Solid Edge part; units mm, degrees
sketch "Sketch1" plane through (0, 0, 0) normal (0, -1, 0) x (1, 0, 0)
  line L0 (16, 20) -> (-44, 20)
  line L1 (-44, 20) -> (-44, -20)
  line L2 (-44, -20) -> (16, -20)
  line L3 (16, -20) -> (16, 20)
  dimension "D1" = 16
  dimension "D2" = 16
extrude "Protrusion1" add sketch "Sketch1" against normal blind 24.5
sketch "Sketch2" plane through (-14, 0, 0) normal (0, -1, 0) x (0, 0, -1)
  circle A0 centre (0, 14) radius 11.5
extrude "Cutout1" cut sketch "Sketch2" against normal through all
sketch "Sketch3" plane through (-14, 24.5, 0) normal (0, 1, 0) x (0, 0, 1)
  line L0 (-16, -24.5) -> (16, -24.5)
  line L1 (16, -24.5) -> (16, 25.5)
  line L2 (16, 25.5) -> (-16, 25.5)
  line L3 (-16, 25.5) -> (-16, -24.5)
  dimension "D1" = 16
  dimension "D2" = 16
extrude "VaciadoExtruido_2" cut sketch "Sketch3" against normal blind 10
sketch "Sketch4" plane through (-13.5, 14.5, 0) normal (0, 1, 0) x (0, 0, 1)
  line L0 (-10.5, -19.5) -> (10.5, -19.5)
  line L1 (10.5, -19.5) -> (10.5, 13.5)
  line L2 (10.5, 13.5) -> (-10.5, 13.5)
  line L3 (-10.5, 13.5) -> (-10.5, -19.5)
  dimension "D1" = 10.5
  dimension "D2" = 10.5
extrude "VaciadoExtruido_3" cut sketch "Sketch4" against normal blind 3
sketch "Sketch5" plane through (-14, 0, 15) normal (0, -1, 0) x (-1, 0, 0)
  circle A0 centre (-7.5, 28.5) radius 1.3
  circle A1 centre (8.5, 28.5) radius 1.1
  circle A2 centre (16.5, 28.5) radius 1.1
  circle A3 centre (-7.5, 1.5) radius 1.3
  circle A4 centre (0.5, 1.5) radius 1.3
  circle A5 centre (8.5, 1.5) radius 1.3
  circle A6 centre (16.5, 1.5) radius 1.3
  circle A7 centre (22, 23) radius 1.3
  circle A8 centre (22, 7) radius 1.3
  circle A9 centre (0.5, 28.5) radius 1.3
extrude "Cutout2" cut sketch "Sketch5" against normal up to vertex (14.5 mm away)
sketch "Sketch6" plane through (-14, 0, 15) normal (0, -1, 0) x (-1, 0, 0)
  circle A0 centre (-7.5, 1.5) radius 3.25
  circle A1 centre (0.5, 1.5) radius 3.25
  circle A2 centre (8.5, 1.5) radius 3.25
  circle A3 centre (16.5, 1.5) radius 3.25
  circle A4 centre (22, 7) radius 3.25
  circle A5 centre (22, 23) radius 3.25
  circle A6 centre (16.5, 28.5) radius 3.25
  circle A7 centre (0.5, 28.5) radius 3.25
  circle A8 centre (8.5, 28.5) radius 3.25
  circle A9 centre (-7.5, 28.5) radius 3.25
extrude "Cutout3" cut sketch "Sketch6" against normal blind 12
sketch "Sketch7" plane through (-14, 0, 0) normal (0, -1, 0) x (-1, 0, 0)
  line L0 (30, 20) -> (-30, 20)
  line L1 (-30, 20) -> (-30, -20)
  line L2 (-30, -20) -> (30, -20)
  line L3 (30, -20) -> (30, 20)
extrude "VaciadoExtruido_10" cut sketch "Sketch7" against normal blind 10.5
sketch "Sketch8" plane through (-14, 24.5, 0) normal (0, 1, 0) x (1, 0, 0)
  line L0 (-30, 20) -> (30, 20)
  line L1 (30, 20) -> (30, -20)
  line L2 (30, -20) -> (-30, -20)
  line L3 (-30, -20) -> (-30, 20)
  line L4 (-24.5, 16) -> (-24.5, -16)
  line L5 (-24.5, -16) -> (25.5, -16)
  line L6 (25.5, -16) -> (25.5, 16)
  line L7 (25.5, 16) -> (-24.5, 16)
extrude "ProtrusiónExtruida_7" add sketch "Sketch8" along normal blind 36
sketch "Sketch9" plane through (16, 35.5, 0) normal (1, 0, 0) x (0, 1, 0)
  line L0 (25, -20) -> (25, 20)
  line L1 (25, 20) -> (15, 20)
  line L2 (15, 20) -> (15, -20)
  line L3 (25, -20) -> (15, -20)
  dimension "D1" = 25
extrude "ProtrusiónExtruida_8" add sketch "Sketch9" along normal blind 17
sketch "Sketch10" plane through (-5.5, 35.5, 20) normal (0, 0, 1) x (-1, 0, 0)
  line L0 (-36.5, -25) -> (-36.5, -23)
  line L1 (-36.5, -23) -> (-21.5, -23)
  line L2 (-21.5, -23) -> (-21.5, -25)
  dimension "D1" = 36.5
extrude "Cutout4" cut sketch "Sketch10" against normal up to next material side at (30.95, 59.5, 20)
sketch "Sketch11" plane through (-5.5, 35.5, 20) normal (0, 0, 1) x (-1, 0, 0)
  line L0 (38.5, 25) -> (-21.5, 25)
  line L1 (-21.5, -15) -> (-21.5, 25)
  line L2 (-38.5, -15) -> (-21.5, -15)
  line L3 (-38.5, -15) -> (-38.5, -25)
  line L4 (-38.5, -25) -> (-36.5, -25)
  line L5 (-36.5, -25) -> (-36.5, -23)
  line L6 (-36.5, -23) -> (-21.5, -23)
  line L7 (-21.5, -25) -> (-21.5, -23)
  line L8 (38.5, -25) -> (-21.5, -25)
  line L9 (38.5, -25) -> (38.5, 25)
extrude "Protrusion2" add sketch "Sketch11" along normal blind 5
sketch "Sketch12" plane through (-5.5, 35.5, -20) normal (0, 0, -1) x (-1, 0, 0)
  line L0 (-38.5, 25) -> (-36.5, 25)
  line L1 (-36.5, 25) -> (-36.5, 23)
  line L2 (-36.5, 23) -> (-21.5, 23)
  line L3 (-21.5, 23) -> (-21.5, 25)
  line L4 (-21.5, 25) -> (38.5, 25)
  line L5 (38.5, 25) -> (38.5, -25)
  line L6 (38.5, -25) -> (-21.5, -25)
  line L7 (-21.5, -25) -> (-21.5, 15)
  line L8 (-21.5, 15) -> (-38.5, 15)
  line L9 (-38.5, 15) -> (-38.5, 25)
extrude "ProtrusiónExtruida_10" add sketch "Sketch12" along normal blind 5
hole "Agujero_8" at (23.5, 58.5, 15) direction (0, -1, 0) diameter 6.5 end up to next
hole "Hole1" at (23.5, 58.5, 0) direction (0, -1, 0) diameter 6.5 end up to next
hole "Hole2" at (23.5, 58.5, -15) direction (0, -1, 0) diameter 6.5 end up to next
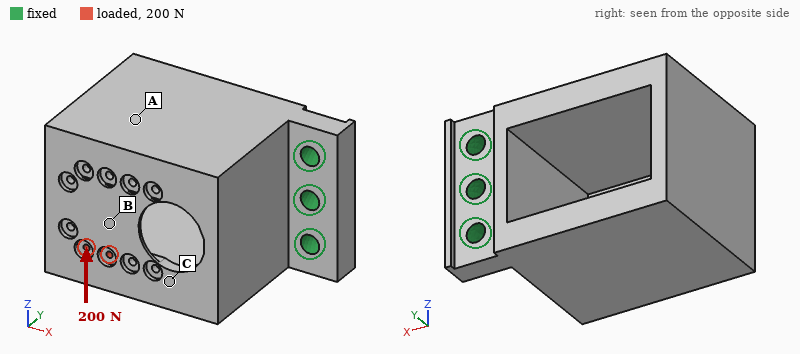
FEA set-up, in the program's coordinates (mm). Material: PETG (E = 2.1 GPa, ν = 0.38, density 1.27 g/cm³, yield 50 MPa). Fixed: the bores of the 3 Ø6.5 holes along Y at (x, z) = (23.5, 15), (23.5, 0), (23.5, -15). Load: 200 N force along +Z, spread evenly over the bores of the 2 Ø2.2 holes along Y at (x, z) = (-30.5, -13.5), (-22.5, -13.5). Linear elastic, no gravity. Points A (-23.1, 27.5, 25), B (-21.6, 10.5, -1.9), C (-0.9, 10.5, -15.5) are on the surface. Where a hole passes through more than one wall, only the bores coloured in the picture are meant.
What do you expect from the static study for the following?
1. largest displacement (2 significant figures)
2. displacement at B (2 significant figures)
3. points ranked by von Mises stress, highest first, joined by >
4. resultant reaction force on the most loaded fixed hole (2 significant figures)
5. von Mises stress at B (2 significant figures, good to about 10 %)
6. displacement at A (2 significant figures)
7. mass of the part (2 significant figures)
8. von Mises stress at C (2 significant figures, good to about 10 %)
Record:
0.50 mm
0.40 mm
B > C > A
340 N
6.0 MPa
0.36 mm
100 g
2.9 MPa
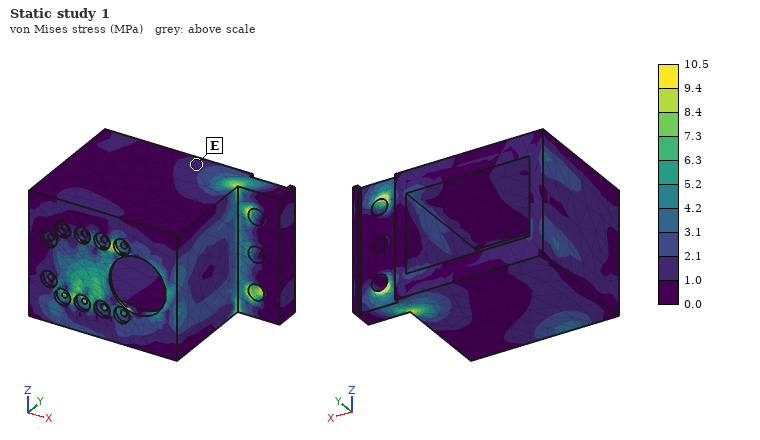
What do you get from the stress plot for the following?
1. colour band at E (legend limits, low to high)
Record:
1.0 to 2.1 MPa
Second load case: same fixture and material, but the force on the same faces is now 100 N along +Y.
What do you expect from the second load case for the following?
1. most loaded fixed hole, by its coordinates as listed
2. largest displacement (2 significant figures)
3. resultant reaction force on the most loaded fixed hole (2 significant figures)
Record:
(23.5, 0)
1.0 mm
70 N
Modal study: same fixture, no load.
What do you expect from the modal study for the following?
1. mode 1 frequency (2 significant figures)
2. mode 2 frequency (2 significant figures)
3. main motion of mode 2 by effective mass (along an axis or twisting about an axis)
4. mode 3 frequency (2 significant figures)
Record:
210 Hz
420 Hz
along Z
820 Hz
